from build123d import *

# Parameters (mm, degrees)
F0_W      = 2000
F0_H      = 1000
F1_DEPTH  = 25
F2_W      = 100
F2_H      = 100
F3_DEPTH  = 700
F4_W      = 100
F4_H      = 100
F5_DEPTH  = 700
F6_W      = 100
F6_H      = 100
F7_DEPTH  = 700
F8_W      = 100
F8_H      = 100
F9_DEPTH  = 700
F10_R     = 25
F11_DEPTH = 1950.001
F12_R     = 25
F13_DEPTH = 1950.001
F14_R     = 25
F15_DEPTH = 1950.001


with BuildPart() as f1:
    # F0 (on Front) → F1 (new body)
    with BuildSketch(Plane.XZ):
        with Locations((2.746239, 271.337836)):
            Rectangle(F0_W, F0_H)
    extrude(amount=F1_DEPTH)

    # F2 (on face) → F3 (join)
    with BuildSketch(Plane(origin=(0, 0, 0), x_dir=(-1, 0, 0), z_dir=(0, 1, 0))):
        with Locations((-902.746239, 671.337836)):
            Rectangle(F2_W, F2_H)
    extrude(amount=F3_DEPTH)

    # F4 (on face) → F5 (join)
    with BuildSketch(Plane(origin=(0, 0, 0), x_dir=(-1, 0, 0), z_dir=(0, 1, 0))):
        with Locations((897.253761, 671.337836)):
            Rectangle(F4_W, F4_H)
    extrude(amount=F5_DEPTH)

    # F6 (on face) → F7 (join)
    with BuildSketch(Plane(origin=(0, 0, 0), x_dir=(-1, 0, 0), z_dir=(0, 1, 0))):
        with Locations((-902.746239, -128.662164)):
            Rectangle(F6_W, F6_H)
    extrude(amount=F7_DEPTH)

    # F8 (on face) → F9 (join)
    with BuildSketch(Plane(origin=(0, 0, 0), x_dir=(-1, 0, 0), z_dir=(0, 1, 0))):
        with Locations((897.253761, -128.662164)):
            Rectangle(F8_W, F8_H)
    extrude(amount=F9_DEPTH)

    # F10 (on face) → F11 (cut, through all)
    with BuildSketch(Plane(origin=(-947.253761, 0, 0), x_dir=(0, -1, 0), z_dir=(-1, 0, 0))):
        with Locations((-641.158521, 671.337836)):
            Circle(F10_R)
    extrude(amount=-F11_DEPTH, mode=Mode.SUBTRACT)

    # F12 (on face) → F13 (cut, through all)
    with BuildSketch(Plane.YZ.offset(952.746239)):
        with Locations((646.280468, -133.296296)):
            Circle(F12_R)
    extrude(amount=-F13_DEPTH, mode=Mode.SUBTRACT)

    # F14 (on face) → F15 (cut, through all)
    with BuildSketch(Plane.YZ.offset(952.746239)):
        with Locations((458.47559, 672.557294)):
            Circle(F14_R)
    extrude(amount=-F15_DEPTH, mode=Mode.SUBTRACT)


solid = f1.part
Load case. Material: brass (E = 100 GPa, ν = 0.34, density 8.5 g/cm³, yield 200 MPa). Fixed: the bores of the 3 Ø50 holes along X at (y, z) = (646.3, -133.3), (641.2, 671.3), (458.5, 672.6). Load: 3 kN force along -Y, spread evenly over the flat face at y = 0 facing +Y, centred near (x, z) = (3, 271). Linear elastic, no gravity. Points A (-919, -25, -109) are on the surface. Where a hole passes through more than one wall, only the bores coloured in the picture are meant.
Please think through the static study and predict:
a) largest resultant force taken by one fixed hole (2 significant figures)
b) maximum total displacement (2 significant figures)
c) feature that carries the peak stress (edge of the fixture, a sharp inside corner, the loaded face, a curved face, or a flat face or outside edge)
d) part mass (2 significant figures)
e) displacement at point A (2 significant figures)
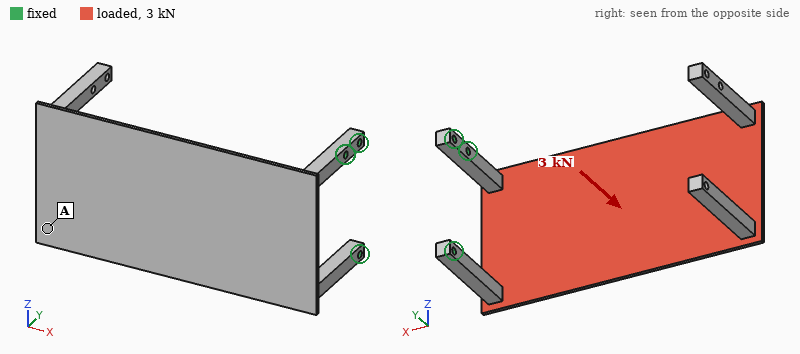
1.8 kN
22 mm
a flat face or outside edge
650 kg
19 mm
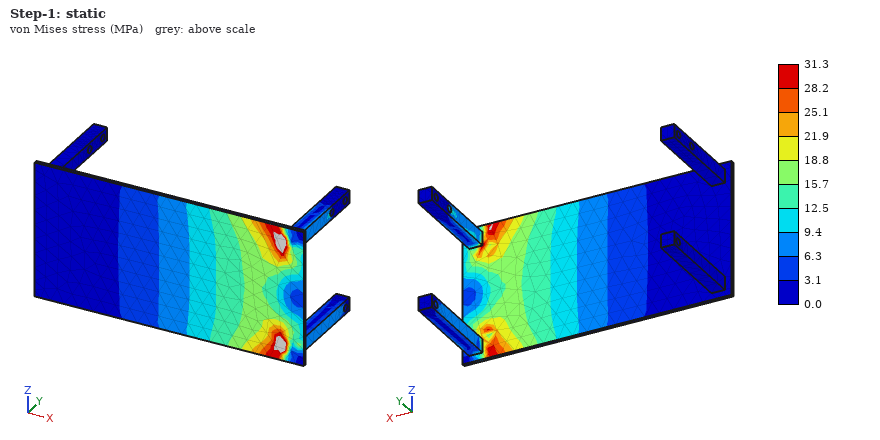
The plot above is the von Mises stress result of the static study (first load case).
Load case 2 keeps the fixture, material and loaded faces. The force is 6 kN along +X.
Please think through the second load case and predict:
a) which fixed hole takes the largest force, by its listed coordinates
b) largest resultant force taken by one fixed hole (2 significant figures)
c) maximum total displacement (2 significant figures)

(458.5, 672.6)
3.8 kN
0.58 mm
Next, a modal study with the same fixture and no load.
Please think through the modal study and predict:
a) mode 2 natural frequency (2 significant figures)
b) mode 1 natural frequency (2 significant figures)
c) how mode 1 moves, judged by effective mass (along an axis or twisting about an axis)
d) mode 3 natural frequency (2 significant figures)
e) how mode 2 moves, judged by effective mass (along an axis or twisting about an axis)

7.7 Hz
2.6 Hz
along Y
13 Hz
along Z
